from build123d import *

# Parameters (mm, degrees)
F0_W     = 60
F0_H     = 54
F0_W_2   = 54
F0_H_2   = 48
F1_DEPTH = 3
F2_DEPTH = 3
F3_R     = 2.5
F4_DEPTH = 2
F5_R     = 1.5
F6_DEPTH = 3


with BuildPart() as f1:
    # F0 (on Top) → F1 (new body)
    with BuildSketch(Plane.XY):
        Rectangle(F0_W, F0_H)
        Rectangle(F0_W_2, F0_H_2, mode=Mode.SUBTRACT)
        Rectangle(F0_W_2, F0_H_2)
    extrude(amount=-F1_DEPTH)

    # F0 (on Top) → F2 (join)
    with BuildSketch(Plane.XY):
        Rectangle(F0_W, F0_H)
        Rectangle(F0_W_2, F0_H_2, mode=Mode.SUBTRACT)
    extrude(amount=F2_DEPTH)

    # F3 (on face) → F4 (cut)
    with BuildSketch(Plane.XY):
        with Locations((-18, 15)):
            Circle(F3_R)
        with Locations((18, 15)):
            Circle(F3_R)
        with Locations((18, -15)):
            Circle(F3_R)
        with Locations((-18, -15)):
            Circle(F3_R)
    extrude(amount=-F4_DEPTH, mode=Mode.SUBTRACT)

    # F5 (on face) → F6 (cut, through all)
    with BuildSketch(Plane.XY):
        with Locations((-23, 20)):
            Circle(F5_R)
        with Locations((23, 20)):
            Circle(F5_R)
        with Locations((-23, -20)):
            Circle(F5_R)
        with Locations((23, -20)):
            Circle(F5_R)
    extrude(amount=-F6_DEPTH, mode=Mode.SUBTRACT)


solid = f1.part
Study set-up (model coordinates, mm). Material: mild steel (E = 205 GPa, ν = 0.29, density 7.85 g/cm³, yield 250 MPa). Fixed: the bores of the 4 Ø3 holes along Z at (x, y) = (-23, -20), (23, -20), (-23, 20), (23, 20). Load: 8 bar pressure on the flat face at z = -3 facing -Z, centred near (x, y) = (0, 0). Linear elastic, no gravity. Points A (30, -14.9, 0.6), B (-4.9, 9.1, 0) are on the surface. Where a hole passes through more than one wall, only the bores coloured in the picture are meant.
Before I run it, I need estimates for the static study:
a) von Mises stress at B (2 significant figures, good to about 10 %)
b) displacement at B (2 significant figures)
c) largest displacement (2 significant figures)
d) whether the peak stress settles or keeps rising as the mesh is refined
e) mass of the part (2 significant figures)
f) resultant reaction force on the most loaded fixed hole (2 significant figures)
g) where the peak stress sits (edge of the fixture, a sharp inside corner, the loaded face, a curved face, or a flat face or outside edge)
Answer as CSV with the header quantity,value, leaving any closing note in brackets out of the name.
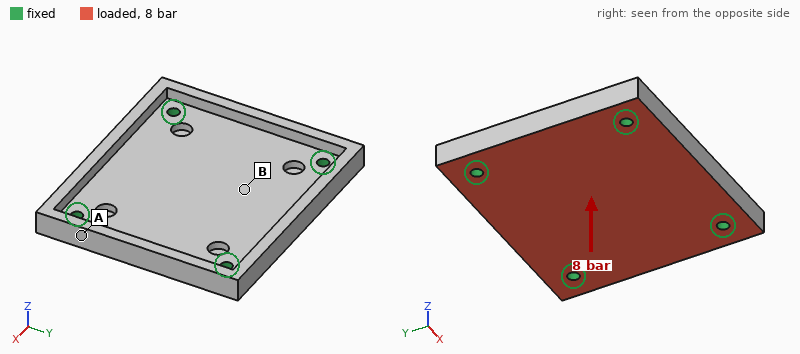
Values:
quantity,value
von Mises stress at B,39 MPa
displacement at B,30 µm
largest displacement,36 µm
whether the peak stress settles or keeps rising as the mesh is refined,keeps rising
mass of the part,90 g
resultant reaction force on the most loaded fixed hole,650 N
where the peak stress sits,edge of the fixture
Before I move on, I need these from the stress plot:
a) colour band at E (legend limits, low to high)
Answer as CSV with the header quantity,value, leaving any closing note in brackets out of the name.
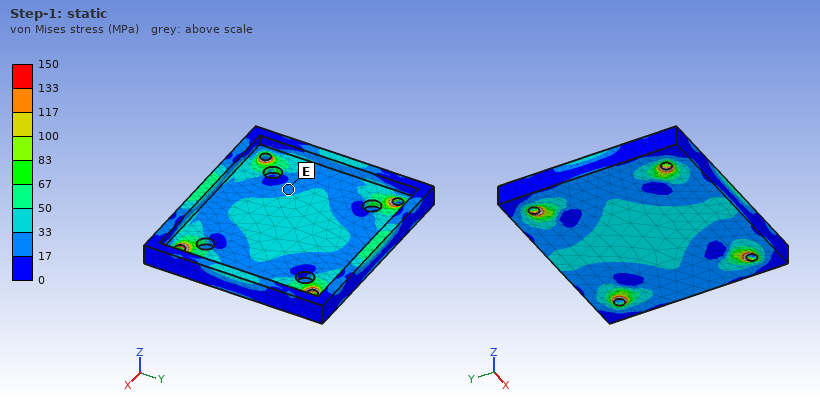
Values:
quantity,value
colour band at E,17 to 33 MPa
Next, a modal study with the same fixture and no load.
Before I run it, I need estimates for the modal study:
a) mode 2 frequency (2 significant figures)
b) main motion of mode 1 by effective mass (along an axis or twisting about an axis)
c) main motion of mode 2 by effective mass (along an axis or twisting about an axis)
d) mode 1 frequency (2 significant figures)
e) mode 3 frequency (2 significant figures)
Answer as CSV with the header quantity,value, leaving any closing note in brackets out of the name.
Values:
quantity,value
mode 2 frequency,9200 Hz
main motion of mode 1 by effective mass,along Z
main motion of mode 2 by effective mass,twisting about X
mode 1 frequency,6000 Hz
mode 3 frequency,10 kHz
